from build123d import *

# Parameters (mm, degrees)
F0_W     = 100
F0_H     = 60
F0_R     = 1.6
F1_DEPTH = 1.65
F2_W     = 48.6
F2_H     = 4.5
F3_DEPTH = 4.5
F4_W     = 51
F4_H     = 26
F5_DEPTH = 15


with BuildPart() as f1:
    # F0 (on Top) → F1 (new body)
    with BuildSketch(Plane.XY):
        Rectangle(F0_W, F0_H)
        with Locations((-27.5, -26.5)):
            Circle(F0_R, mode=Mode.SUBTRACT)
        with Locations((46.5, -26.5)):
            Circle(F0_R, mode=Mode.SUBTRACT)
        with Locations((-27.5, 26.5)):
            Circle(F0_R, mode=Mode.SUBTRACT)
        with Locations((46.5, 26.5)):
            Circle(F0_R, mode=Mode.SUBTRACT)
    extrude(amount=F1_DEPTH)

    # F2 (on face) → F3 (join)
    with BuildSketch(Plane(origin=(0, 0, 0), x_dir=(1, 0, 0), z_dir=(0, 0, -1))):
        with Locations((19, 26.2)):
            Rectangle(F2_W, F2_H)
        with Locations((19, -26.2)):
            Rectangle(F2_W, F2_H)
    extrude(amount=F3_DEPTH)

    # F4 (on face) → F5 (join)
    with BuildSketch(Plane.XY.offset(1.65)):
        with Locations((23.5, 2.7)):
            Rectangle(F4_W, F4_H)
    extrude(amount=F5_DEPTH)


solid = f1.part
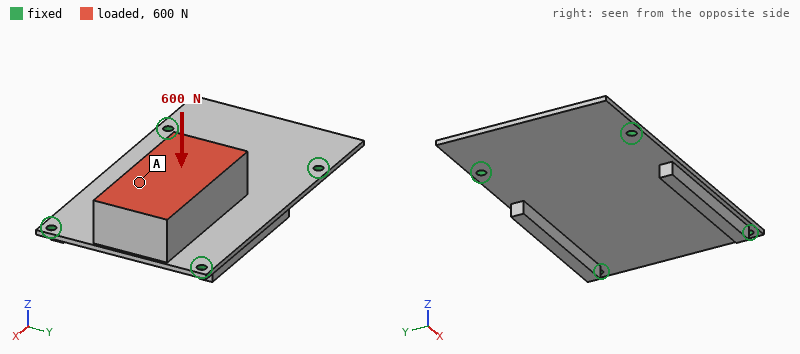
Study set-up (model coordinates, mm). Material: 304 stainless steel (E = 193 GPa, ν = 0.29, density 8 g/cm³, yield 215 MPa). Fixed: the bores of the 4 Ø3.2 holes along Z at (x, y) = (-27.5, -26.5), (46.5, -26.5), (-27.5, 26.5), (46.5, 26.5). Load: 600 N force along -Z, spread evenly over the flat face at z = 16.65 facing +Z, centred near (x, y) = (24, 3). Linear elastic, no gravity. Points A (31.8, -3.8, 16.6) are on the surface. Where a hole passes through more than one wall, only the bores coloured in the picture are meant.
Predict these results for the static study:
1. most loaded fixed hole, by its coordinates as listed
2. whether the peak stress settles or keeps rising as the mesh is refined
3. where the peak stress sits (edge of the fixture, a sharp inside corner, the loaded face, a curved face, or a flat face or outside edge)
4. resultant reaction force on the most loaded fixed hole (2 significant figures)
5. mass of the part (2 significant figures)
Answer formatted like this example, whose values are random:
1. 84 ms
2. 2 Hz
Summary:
1. (46.5, 26.5)
2. keeps rising
3. edge of the fixture
4. 270 N
5. 250 g
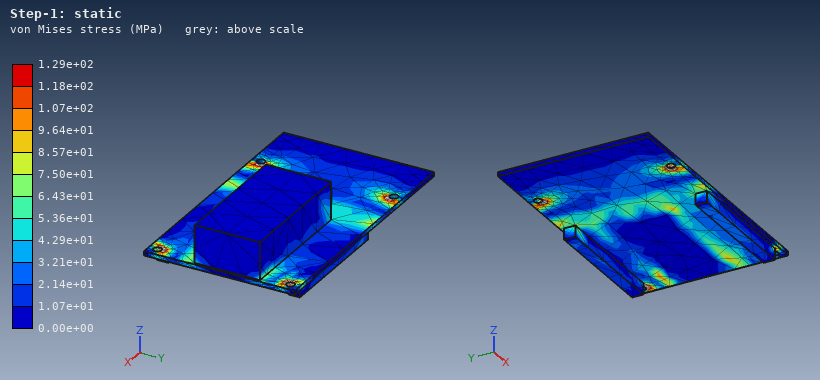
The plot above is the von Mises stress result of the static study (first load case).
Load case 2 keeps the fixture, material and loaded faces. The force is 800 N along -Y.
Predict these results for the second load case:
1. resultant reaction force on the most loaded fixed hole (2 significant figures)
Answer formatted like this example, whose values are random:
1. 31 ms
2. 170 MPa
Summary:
1. 360 N
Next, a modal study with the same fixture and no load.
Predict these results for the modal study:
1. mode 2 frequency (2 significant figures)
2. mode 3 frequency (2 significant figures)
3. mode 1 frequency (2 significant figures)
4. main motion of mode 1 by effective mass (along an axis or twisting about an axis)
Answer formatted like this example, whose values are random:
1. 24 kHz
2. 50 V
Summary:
1. 1800 Hz
2. 1900 Hz
3. 1000 Hz
4. along Z
